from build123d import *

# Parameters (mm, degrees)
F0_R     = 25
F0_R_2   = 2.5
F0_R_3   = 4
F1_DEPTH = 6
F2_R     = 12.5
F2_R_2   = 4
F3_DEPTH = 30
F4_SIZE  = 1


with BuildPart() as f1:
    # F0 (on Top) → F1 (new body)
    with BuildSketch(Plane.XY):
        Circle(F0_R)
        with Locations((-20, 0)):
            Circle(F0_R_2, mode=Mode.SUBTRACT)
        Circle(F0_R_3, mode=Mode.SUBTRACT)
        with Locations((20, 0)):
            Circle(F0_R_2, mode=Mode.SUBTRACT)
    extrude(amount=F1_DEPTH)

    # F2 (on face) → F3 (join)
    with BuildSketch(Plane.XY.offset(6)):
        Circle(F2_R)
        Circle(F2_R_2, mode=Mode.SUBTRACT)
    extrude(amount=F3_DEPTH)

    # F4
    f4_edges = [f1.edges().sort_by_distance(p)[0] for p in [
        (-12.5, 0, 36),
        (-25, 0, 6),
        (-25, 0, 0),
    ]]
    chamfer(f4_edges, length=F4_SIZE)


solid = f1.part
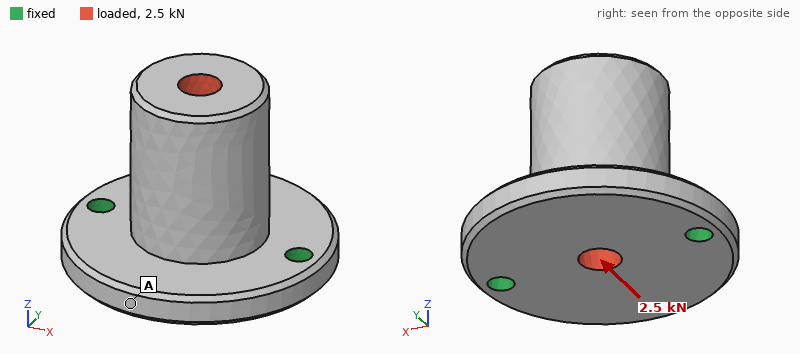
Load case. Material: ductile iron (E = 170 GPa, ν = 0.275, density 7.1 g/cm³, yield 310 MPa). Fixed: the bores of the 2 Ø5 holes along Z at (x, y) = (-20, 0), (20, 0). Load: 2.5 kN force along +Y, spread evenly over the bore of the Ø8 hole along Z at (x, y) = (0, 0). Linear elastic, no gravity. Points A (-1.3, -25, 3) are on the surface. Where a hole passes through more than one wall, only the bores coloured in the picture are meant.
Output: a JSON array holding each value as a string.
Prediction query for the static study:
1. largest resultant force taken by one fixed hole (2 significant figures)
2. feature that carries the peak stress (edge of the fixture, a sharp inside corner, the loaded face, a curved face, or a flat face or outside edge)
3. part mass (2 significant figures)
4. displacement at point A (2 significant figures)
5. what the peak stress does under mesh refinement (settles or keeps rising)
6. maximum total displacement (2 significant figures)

["1.3 kN", "edge of the fixture", "170 g", "39 µm", "keeps rising", "61 µm"]
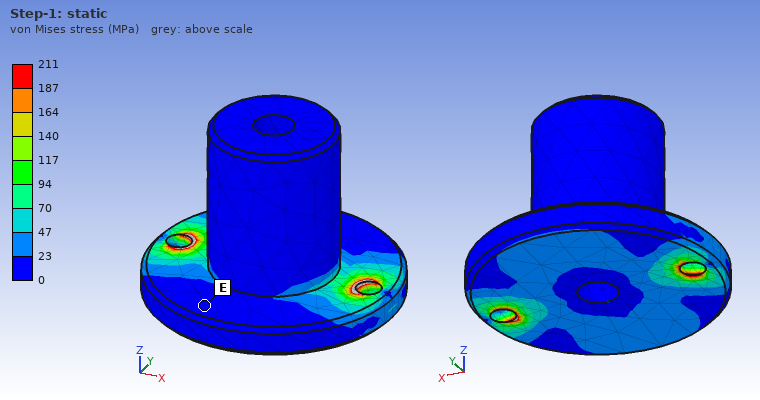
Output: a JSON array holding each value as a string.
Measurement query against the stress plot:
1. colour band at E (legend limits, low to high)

["0 to 23 MPa"]
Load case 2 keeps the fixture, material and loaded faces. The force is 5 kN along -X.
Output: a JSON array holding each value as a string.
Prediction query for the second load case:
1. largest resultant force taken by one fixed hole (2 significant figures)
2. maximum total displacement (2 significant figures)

["3.4 kN", "24 µm"]
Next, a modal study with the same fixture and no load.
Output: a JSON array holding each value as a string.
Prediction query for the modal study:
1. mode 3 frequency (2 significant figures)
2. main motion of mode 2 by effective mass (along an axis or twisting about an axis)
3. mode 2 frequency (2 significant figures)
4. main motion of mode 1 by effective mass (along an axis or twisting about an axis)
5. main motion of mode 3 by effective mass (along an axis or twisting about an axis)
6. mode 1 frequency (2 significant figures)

["9300 Hz", "along X", "8100 Hz", "along Y", "along Z", "3300 Hz"]
